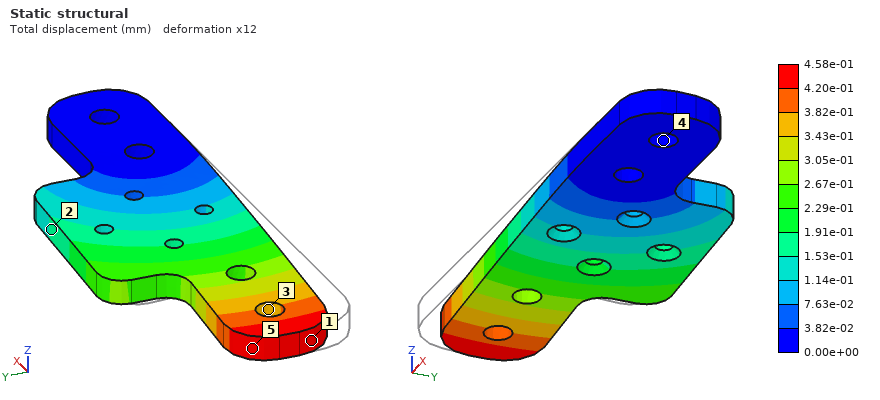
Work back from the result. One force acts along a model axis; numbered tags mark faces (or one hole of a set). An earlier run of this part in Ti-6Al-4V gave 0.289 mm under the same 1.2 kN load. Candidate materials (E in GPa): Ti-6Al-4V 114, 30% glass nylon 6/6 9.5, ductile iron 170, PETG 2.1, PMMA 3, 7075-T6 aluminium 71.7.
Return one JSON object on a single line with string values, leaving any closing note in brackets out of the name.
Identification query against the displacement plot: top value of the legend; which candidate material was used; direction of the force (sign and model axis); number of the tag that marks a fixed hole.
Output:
{"top value of the legend": "4.58e-01 mm", "which candidate material was used": "7075-T6 aluminium", "direction of the force": "+Y", "number of the tag that marks a fixed hole": "4"}
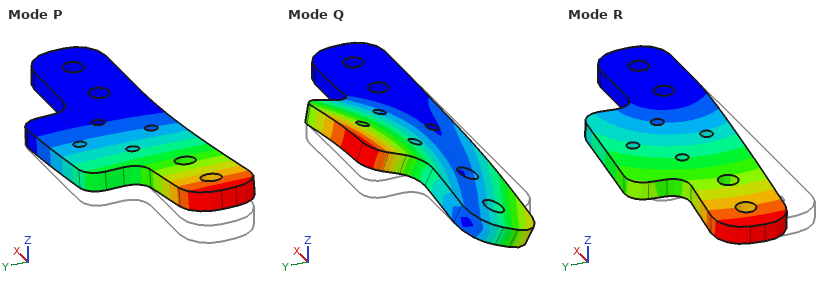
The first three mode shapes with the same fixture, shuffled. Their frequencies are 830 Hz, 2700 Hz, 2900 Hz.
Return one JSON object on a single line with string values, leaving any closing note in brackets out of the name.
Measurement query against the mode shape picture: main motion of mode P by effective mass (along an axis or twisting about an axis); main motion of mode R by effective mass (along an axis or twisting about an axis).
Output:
{"main motion of mode P by effective mass": "along Z", "main motion of mode R by effective mass": "along Y"}
